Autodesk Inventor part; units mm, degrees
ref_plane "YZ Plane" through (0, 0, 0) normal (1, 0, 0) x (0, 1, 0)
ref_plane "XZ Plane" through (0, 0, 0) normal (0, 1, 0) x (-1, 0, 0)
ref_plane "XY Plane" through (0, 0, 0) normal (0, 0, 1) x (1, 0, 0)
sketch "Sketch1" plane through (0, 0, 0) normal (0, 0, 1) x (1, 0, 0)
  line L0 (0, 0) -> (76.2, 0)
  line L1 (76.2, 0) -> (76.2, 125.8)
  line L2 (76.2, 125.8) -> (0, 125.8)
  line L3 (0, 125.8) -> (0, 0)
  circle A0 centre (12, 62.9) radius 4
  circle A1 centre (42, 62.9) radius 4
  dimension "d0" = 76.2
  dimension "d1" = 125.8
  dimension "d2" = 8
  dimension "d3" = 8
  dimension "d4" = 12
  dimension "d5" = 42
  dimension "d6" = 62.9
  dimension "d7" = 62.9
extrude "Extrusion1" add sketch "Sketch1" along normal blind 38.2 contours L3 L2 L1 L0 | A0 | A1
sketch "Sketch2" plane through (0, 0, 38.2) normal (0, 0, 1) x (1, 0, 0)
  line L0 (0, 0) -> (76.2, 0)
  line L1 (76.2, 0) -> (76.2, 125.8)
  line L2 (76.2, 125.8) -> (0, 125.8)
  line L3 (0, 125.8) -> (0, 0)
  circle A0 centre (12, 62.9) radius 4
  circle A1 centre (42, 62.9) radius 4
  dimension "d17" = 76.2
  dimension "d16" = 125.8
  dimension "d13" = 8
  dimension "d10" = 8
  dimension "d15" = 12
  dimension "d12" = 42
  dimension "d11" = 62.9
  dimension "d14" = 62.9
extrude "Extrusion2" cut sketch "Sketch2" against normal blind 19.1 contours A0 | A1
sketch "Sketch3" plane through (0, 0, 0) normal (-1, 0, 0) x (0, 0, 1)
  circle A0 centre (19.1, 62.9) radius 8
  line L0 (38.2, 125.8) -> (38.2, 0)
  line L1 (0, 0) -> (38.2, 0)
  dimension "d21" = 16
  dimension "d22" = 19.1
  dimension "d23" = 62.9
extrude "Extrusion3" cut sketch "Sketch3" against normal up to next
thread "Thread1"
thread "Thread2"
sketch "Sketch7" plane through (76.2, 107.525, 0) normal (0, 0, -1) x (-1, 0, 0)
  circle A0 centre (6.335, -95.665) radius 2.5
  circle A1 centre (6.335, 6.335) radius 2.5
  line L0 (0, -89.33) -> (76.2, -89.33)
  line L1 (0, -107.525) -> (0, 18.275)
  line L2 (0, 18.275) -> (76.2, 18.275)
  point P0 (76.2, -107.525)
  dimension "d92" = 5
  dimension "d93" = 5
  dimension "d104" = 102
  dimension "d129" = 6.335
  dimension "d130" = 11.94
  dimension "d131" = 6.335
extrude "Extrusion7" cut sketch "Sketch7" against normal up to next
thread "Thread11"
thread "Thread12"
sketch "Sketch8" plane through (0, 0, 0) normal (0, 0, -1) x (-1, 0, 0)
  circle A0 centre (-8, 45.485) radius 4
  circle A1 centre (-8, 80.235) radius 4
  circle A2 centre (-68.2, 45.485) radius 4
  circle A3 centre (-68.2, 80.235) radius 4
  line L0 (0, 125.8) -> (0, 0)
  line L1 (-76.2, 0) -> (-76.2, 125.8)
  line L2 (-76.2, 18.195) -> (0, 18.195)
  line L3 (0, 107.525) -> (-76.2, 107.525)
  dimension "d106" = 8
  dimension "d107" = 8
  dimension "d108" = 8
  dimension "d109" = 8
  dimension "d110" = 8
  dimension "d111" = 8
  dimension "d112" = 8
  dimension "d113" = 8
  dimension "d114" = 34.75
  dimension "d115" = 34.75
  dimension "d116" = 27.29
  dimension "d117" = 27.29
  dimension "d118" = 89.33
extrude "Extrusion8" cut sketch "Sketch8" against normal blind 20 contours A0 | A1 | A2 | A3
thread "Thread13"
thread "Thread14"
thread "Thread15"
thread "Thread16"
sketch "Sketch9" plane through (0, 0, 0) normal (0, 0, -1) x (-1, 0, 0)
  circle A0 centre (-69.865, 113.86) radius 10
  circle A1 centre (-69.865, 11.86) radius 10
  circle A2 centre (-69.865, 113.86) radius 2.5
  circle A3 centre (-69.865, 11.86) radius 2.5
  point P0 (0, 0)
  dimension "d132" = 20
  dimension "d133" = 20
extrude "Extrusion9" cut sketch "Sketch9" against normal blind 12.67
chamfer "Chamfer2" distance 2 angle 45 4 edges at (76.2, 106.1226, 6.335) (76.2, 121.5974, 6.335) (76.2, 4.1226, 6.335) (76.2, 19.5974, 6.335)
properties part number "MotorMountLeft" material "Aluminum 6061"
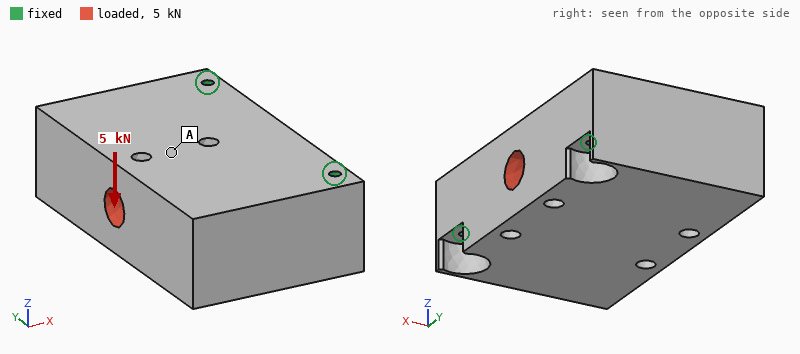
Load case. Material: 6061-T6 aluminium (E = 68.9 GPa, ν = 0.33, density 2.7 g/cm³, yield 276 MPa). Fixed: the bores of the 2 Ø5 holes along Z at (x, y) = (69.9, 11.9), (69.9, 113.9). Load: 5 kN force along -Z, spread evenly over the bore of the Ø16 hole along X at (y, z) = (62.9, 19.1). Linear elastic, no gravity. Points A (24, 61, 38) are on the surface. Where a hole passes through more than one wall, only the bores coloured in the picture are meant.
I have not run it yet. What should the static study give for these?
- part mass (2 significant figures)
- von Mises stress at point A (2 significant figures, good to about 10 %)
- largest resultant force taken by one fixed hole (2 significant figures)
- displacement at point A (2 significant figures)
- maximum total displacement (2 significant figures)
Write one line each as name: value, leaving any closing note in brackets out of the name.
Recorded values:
part mass: 910 g
von Mises stress at point A: 6.1 MPa
largest resultant force taken by one fixed hole: 2.5 kN
displacement at point A: 32 µm
maximum total displacement: 49 µm
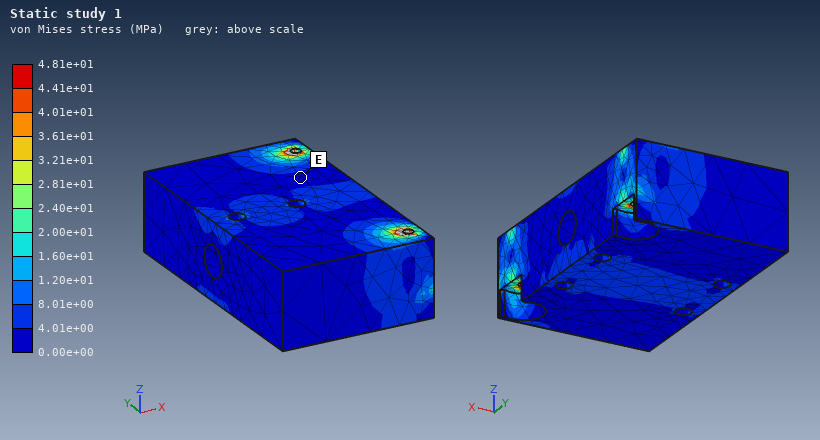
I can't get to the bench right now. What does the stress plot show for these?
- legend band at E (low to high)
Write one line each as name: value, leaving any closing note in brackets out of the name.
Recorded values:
legend band at E: 0.00e+00 to 4.01e+00 MPa
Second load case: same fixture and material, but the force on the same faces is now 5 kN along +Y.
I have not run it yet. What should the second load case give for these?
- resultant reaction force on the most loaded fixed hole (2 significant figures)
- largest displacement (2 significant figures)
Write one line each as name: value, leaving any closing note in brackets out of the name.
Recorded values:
resultant reaction force on the most loaded fixed hole: 2.9 kN
largest displacement: 4.3 µm
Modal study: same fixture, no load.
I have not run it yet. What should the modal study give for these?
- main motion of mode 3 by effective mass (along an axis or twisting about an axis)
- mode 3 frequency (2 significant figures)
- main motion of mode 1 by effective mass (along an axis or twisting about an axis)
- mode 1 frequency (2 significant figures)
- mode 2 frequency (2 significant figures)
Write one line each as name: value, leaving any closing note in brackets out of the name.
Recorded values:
main motion of mode 3 by effective mass: along Y
mode 3 frequency: 6600 Hz
main motion of mode 1 by effective mass: along Z
mode 1 frequency: 2100 Hz
mode 2 frequency: 5400 Hz
